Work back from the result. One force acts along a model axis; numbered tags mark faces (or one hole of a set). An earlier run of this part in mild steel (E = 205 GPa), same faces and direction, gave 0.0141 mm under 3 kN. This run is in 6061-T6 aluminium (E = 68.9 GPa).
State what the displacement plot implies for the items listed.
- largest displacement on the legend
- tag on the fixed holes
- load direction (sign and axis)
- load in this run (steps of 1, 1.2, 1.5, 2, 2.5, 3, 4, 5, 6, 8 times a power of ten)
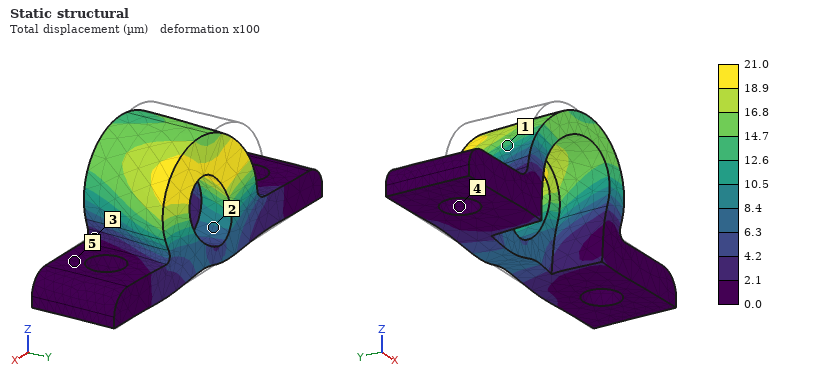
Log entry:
21.0 µm
4
+X
1.5 kN
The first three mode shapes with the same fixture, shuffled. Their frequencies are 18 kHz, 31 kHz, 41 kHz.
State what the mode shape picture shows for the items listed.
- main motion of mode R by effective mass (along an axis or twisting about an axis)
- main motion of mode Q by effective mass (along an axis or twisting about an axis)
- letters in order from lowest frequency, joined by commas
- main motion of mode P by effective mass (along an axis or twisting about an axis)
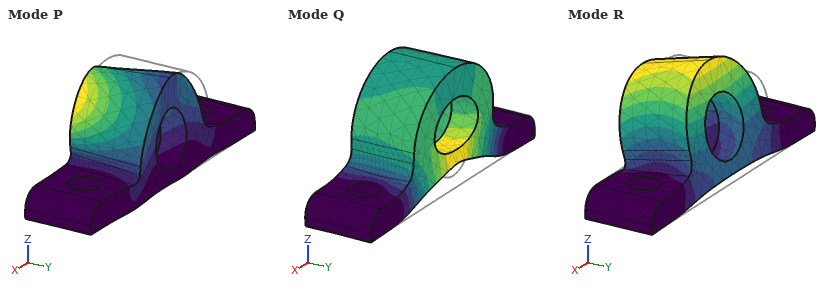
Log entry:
along Y
along Z
R, P, Q
along X
